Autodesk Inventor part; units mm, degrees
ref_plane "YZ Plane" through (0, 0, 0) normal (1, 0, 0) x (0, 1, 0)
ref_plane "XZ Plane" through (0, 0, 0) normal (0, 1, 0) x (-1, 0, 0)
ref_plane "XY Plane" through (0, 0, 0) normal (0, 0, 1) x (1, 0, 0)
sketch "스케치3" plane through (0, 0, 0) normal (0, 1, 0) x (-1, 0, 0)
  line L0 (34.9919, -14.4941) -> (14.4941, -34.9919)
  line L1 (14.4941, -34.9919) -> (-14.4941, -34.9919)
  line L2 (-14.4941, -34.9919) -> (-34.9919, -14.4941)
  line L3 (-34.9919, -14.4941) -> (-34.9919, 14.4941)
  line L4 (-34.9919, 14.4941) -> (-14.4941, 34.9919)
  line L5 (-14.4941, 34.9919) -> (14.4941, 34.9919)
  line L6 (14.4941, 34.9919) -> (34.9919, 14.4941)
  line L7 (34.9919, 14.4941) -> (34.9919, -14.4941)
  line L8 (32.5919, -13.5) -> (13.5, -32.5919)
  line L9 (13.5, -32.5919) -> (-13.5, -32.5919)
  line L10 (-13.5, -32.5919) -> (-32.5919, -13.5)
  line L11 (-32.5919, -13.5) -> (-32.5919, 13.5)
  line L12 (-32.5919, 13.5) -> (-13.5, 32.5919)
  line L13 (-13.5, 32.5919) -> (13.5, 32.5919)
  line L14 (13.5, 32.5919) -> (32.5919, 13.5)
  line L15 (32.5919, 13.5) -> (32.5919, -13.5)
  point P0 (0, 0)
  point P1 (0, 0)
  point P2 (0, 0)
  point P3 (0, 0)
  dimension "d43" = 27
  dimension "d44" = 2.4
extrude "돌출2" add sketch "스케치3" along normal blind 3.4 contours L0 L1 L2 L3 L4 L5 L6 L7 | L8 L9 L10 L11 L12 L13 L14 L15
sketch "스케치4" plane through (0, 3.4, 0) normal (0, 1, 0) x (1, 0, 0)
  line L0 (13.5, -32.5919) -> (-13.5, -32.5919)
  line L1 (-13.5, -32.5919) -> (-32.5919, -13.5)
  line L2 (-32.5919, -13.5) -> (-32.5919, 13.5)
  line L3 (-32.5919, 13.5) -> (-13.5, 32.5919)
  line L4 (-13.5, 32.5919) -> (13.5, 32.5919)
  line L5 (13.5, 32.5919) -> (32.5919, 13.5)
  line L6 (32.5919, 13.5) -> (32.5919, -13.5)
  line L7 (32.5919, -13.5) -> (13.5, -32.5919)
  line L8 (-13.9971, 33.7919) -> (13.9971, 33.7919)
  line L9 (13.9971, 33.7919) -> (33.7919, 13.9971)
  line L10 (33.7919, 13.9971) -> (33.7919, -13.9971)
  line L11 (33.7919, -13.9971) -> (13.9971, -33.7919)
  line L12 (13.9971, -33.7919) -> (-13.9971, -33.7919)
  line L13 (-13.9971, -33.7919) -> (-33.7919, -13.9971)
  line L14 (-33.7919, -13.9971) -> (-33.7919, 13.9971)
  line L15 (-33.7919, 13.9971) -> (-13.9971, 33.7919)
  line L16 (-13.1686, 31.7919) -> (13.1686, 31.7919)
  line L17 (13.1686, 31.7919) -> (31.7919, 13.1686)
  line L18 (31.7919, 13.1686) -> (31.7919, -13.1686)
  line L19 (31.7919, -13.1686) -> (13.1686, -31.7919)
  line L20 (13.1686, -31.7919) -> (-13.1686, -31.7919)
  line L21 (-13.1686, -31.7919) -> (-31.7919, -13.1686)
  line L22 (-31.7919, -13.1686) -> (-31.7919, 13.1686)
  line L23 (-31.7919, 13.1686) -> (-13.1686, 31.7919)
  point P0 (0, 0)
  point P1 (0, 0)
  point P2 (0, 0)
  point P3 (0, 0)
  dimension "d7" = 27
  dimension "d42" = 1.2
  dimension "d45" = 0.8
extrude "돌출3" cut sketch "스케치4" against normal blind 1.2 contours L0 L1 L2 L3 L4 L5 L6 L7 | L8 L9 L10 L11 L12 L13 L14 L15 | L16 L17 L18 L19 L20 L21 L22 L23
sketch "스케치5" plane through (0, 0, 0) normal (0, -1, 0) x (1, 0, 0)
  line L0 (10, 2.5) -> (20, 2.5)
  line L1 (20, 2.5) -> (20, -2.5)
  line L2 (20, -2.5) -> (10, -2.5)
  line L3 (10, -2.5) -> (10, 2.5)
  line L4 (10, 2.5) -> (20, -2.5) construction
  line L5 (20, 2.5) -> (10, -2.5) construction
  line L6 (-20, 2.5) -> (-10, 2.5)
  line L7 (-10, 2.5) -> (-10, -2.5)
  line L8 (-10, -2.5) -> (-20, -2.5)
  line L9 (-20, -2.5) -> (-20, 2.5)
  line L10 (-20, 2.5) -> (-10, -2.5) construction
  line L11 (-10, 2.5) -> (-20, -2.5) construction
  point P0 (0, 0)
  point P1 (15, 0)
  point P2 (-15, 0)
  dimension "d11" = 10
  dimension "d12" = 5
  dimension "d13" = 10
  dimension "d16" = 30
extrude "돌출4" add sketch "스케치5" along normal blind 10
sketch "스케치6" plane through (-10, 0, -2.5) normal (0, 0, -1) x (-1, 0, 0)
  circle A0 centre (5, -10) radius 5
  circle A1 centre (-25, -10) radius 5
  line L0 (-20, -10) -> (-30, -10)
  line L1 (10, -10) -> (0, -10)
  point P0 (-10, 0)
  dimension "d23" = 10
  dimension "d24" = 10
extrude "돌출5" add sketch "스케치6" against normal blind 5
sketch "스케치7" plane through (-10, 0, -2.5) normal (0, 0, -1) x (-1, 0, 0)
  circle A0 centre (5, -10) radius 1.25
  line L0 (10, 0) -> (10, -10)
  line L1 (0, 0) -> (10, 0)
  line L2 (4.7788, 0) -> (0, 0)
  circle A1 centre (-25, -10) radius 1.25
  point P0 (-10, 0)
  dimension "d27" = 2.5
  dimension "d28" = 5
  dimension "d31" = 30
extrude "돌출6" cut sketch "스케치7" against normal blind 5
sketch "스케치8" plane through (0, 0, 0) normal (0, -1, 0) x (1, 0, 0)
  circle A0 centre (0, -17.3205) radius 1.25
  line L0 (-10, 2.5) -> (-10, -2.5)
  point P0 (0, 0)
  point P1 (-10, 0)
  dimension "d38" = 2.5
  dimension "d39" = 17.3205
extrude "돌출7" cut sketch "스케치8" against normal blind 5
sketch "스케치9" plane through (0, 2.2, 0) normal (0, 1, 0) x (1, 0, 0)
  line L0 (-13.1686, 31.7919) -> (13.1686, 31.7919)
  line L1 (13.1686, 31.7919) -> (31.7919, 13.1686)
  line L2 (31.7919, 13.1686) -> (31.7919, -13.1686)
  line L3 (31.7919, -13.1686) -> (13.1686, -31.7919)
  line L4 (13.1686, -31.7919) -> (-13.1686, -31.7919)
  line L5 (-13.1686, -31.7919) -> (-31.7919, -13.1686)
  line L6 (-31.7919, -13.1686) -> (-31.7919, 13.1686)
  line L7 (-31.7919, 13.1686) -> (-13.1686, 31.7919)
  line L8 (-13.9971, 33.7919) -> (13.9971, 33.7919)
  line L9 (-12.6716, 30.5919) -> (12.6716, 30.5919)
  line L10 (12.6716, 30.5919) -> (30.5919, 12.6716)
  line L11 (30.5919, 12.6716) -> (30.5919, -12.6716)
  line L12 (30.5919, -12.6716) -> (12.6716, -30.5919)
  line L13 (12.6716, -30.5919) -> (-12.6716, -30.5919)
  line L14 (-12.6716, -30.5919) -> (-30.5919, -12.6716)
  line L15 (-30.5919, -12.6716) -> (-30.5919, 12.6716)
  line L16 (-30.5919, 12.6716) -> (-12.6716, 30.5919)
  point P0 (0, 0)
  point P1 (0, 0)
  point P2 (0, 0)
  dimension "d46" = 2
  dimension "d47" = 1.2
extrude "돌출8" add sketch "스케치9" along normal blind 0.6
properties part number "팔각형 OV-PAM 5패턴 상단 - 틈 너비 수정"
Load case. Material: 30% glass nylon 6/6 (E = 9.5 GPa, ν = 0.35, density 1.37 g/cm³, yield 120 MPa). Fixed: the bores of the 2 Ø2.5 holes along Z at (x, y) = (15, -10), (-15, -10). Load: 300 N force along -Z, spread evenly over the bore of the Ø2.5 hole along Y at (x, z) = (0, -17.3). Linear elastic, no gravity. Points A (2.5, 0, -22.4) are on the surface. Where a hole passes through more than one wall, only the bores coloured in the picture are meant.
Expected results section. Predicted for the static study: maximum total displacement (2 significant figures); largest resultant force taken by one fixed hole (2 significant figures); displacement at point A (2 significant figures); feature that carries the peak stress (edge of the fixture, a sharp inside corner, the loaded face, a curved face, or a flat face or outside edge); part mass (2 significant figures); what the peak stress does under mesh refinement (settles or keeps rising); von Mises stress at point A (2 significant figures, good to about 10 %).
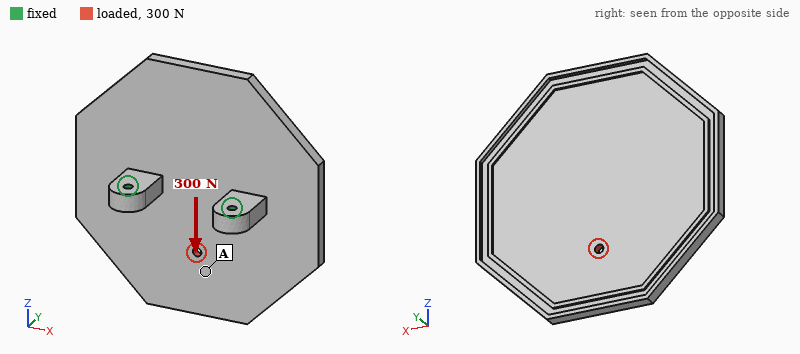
0.37 mm
150 N
0.24 mm
edge of the fixture
15 g
keeps rising
5.5 MPa
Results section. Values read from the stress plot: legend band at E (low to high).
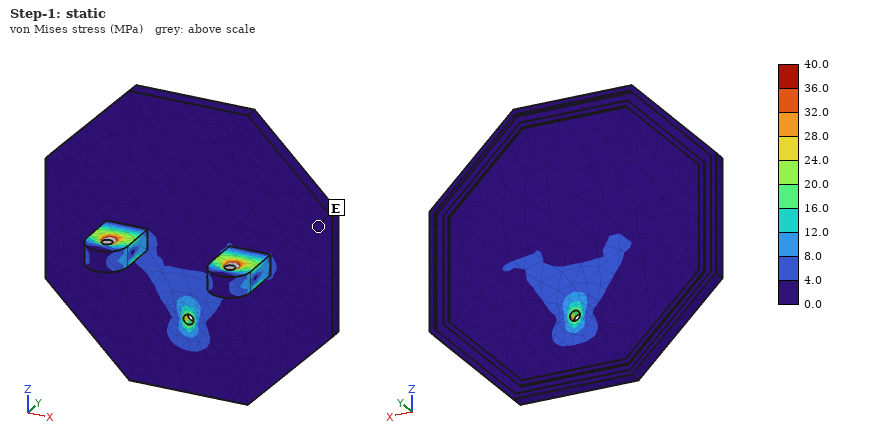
0.0 to 4.0 MPa
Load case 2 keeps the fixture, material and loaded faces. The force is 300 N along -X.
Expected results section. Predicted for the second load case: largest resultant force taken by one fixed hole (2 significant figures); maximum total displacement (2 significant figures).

210 N
0.24 mm
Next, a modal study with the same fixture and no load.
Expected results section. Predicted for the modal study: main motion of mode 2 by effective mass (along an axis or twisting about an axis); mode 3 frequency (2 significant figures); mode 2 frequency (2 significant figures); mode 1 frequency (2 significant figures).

along Y
1400 Hz
1000 Hz
680 Hz
